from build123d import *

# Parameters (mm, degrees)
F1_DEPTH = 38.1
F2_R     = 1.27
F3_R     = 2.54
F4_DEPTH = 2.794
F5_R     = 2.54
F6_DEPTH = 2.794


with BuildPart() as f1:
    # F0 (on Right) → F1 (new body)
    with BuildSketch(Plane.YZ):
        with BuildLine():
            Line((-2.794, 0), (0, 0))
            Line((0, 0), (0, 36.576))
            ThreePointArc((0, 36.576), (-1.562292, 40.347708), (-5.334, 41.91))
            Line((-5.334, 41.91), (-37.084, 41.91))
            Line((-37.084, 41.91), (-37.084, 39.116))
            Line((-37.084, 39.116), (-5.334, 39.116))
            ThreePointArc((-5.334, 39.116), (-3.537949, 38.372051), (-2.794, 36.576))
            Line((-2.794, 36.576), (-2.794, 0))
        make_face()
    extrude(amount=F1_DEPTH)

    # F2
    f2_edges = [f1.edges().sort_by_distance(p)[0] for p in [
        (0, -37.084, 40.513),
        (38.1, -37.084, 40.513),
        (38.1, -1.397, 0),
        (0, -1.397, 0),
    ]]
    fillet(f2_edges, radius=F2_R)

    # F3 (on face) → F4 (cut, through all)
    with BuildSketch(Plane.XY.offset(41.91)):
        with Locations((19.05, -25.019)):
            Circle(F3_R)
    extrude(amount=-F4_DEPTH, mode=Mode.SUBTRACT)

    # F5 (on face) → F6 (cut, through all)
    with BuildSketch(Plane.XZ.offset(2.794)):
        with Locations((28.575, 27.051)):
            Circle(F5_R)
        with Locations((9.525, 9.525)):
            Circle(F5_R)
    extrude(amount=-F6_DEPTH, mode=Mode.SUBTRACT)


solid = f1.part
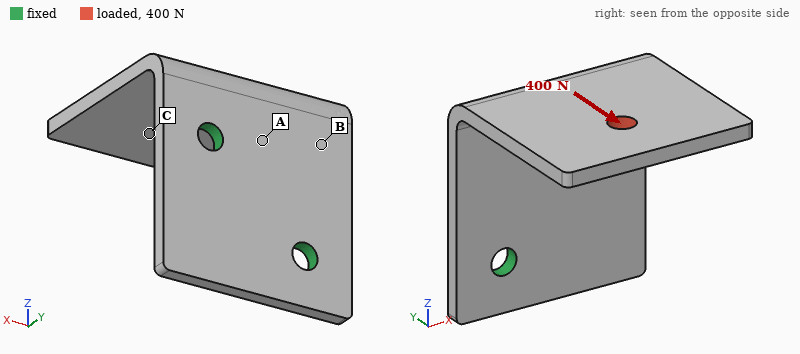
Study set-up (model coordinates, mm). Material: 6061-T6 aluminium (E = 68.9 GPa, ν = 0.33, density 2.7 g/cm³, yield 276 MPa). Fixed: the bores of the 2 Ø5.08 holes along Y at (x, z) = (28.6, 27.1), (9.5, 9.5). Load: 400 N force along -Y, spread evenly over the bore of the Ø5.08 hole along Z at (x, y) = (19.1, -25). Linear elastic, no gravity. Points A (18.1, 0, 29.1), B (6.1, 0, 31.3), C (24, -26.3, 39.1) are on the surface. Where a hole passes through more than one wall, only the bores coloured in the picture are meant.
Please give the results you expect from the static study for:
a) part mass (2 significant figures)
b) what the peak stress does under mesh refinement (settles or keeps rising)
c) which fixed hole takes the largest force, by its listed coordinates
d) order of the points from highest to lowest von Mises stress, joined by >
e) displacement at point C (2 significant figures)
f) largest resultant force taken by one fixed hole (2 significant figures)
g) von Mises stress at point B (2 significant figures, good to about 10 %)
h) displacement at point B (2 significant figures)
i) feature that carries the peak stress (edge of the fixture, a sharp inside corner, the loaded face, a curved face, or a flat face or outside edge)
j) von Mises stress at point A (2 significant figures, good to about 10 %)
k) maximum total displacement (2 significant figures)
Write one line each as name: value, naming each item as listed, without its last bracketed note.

part mass: 21 g
what the peak stress does under mesh refinement: keeps rising
which fixed hole takes the largest force, by its listed coordinates: (28.6, 27.1)
order of the points from highest to lowest von Mises stress, joined by >: A > B > C
displacement at point C: 0.28 mm
largest resultant force taken by one fixed hole: 390 N
von Mises stress at point B: 37 MPa
displacement at point B: 0.10 mm
feature that carries the peak stress: edge of the fixture
von Mises stress at point A: 67 MPa
maximum total displacement: 0.47 mm
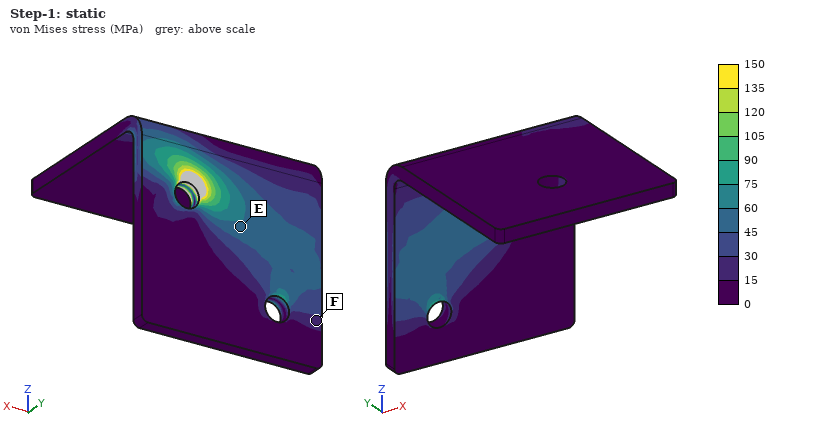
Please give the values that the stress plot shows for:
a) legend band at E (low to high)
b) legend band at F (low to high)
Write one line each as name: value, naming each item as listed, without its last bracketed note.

legend band at E: 45 to 60 MPa
legend band at F: 15 to 30 MPa
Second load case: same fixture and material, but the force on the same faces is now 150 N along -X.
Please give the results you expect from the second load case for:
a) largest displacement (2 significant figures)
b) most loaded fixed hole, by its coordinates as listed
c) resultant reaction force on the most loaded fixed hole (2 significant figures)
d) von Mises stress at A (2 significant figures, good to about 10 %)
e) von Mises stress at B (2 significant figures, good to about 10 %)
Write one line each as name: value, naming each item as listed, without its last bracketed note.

largest displacement: 0.25 mm
most loaded fixed hole, by its coordinates as listed: (28.6, 27.1)
resultant reaction force on the most loaded fixed hole: 180 N
von Mises stress at A: 28 MPa
von Mises stress at B: 22 MPa
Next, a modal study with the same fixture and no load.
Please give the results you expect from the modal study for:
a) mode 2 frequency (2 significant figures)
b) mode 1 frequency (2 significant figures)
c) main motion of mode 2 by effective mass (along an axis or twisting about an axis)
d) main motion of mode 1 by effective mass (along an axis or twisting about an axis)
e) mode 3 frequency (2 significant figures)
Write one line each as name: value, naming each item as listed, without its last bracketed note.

mode 2 frequency: 1800 Hz
mode 1 frequency: 1100 Hz
main motion of mode 2 by effective mass: along X
main motion of mode 1 by effective mass: along Z
mode 3 frequency: 3700 Hz
